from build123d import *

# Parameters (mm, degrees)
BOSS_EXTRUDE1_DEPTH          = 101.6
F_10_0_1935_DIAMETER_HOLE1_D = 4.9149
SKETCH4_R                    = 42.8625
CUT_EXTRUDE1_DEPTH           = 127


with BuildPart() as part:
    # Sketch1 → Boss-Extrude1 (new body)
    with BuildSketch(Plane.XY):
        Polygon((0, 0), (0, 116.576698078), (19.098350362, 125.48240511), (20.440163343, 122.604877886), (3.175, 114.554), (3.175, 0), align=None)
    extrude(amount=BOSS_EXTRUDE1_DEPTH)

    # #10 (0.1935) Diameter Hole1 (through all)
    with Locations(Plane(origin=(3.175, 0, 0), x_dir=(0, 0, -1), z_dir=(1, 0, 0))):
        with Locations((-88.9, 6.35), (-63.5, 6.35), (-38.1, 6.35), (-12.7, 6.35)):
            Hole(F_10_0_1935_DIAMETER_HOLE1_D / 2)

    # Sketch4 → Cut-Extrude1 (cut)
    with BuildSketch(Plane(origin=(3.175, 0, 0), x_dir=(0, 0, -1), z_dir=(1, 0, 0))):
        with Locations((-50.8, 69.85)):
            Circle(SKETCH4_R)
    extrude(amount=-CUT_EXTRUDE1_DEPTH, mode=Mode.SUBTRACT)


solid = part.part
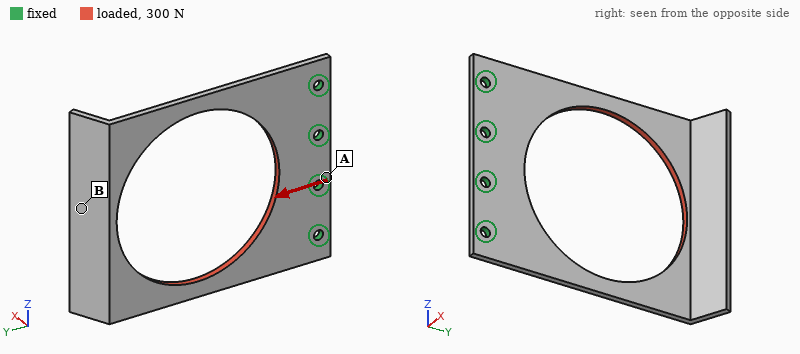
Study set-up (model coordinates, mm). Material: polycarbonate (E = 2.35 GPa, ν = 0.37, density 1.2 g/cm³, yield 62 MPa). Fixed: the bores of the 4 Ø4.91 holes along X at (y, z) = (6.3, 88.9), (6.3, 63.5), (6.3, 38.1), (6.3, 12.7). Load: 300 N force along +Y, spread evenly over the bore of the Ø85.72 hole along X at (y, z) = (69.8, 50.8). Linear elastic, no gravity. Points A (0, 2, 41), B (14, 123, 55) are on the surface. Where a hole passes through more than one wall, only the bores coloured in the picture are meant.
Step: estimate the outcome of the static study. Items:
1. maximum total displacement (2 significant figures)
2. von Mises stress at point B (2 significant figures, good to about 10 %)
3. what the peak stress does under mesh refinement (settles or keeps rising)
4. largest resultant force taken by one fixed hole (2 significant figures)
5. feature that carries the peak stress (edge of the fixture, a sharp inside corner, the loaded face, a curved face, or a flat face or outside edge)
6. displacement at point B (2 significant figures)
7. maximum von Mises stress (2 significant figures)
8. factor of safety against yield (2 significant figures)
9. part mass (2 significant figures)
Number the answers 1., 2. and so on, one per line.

1. 0.68 mm
2. 3.1 MPa
3. settles
4. 160 N
5. the loaded face
6. 0.58 mm
7. 12 MPa
8. 5.3
9. 30 g
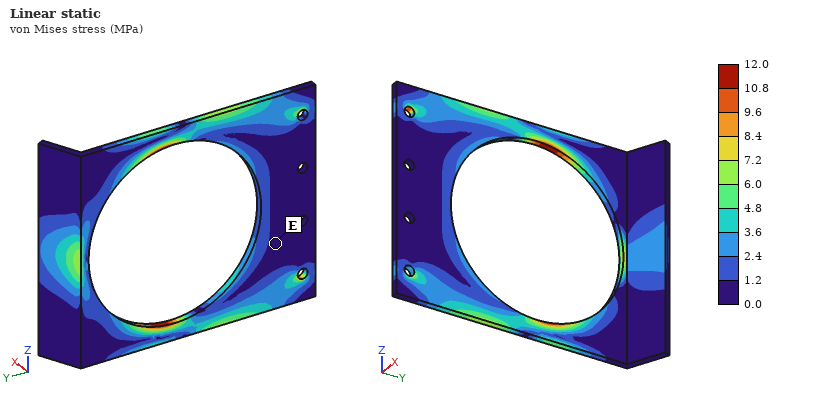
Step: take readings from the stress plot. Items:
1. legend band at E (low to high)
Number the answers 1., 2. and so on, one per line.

1. 0.0 to 1.2 MPa
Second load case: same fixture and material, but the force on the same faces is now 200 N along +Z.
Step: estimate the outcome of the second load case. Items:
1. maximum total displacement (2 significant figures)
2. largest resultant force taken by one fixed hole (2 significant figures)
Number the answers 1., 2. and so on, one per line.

1. 1.8 mm
2. 180 N
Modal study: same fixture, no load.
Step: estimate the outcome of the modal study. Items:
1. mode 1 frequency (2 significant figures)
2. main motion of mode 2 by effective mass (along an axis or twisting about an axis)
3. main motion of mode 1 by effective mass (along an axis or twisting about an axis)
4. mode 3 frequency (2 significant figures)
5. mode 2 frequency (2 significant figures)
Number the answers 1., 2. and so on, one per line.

1. 33 Hz
2. twisting about Y
3. along X
4. 270 Hz
5. 93 Hz
